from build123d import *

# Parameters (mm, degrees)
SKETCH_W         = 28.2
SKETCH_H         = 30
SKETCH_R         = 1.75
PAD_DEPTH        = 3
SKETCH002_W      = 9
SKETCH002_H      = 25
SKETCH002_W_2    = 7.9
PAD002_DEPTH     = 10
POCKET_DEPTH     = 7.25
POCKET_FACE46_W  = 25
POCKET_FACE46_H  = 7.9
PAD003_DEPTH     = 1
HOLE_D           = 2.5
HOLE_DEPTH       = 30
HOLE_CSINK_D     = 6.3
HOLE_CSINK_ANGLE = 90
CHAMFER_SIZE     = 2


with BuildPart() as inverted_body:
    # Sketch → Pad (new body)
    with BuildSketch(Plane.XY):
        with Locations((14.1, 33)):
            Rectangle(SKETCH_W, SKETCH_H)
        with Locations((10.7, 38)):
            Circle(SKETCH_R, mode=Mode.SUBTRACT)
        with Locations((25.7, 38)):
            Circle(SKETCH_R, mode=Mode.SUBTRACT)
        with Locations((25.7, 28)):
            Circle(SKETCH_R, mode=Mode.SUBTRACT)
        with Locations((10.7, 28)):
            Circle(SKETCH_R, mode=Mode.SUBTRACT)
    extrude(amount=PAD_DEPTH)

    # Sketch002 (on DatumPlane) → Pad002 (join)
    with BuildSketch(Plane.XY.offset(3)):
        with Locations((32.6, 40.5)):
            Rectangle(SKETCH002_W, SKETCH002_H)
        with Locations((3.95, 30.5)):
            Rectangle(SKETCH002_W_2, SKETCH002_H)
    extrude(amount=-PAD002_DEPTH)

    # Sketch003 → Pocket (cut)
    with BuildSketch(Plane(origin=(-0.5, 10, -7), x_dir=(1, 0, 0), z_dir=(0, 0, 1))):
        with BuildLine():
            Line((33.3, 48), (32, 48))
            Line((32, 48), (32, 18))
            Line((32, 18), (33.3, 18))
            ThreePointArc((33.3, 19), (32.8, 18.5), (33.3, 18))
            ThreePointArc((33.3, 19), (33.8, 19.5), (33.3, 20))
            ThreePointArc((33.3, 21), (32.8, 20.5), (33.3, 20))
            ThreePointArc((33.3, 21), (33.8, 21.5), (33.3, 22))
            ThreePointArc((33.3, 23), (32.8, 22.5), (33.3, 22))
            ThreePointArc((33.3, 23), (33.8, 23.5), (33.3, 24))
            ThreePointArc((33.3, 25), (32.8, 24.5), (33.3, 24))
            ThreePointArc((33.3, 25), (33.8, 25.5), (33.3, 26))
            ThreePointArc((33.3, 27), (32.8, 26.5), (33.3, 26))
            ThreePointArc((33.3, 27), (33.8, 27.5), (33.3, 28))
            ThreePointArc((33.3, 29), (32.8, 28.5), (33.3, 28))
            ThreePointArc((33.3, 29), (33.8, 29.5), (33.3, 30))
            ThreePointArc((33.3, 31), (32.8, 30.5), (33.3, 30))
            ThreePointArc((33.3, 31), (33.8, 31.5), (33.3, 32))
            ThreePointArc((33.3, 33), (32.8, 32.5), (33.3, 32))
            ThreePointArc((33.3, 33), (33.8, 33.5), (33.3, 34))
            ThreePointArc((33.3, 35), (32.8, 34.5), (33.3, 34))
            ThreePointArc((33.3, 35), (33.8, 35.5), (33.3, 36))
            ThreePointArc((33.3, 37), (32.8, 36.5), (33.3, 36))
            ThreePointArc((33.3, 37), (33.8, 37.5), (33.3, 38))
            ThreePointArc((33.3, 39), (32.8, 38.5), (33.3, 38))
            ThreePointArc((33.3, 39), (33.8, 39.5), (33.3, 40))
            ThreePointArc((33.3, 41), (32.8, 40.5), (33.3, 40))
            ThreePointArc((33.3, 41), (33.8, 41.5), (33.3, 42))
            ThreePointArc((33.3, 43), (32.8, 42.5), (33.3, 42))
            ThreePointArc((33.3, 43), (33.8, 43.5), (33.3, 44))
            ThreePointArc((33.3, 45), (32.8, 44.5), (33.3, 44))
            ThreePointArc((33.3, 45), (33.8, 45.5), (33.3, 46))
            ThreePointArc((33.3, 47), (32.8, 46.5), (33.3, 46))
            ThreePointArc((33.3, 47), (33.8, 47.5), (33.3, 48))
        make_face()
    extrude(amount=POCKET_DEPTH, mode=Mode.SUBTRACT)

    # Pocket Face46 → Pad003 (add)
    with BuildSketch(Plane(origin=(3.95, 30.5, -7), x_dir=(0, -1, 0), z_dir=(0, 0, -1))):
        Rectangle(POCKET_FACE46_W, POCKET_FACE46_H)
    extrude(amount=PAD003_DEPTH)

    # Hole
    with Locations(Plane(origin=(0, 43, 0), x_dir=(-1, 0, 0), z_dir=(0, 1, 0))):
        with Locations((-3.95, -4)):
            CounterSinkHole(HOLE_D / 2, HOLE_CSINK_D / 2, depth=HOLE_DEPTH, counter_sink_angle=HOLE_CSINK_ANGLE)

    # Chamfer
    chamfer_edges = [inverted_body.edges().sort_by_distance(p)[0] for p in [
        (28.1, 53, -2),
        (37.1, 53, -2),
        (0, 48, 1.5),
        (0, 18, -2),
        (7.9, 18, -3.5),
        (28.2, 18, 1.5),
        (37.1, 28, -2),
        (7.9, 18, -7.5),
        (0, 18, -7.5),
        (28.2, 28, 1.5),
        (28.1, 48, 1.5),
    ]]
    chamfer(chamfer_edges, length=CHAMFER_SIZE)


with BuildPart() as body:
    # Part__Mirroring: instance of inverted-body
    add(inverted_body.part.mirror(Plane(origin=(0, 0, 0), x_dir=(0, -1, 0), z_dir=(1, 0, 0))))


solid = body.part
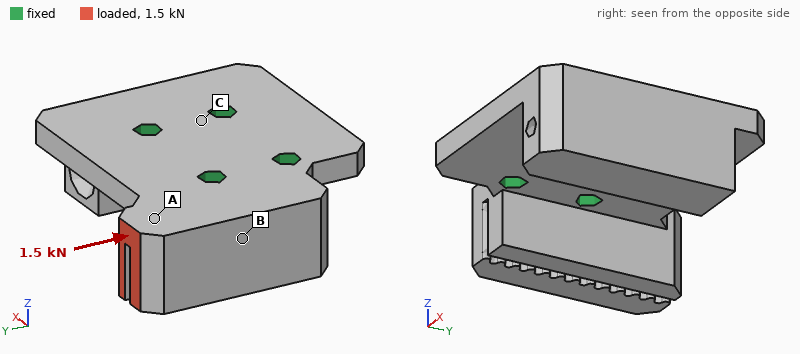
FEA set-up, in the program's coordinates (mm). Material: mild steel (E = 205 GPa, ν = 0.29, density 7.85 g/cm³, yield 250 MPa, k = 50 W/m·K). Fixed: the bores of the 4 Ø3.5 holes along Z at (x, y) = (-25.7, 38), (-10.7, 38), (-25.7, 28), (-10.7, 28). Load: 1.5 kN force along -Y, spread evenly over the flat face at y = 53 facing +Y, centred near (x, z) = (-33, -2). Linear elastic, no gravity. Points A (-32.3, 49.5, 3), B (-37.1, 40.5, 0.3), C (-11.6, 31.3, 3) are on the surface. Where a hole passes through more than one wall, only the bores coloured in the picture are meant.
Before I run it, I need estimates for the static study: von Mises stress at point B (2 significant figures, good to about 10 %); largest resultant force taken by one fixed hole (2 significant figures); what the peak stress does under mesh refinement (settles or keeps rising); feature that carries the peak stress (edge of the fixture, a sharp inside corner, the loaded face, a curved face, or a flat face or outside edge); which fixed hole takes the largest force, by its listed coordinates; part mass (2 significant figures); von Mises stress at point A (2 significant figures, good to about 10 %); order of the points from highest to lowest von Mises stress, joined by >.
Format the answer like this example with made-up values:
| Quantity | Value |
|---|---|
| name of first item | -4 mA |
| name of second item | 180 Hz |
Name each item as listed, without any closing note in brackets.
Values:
| Quantity | Value |
|---|---|
| von Mises stress at point B | 21 MPa |
| largest resultant force taken by one fixed hole | 1.2 kN |
| what the peak stress does under mesh refinement | keeps rising |
| feature that carries the peak stress | edge of the fixture |
| which fixed hole takes the largest force, by its listed coordinates | (-25.7, 38) |
| part mass | 45 g |
| von Mises stress at point A | 35 MPa |
| order of the points from highest to lowest von Mises stress, joined by > | A > B > C |
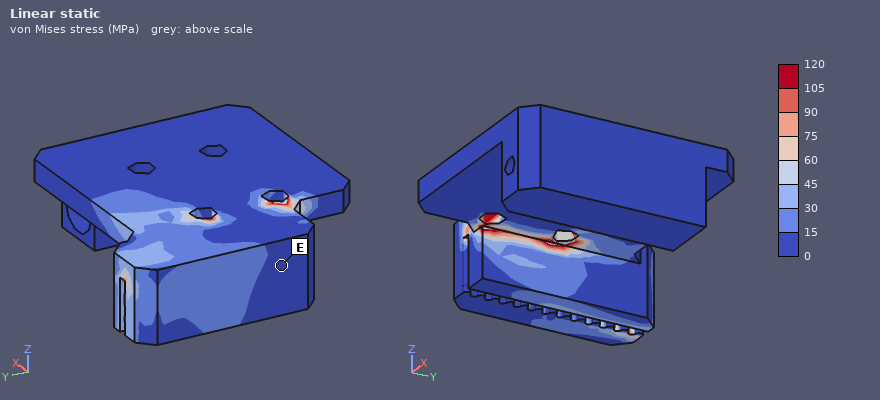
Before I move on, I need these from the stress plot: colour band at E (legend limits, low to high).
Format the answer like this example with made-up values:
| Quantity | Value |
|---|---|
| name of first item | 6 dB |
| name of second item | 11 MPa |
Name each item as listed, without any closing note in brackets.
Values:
| Quantity | Value |
|---|---|
| colour band at E | 0 to 15 MPa |
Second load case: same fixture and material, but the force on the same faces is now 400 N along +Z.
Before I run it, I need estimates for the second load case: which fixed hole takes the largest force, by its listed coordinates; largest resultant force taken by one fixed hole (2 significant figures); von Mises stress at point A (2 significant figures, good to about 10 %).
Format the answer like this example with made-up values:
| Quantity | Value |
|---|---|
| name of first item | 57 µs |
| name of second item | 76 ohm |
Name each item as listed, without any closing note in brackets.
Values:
| Quantity | Value |
|---|---|
| which fixed hole takes the largest force, by its listed coordinates | (-25.7, 38) |
| largest resultant force taken by one fixed hole | 890 N |
| von Mises stress at point A | 22 MPa |
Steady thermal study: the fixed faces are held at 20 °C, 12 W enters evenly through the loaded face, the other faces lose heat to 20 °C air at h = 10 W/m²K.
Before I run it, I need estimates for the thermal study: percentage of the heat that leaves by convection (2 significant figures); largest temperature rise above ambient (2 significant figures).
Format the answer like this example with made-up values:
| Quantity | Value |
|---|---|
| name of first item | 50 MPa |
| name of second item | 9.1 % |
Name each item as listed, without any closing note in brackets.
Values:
| Quantity | Value |
|---|---|
| percentage of the heat that leaves by convection | 3.6 % |
| largest temperature rise above ambient | 68 K |
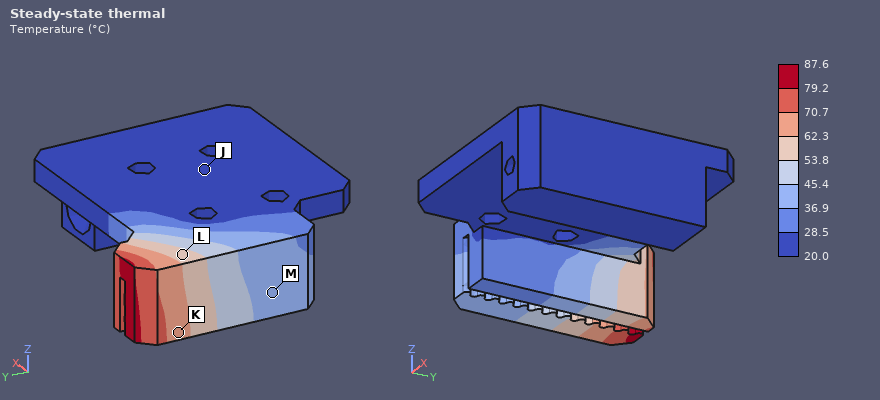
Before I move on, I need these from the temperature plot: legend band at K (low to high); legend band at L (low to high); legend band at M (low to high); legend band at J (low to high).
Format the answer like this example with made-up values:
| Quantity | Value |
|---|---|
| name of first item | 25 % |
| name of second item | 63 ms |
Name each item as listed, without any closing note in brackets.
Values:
| Quantity | Value |
|---|---|
| legend band at K | 62.3 to 70.7 °C |
| legend band at L | 53.8 to 62.3 °C |
| legend band at M | 36.9 to 45.4 °C |
| legend band at J | 20.0 to 28.5 °C |
